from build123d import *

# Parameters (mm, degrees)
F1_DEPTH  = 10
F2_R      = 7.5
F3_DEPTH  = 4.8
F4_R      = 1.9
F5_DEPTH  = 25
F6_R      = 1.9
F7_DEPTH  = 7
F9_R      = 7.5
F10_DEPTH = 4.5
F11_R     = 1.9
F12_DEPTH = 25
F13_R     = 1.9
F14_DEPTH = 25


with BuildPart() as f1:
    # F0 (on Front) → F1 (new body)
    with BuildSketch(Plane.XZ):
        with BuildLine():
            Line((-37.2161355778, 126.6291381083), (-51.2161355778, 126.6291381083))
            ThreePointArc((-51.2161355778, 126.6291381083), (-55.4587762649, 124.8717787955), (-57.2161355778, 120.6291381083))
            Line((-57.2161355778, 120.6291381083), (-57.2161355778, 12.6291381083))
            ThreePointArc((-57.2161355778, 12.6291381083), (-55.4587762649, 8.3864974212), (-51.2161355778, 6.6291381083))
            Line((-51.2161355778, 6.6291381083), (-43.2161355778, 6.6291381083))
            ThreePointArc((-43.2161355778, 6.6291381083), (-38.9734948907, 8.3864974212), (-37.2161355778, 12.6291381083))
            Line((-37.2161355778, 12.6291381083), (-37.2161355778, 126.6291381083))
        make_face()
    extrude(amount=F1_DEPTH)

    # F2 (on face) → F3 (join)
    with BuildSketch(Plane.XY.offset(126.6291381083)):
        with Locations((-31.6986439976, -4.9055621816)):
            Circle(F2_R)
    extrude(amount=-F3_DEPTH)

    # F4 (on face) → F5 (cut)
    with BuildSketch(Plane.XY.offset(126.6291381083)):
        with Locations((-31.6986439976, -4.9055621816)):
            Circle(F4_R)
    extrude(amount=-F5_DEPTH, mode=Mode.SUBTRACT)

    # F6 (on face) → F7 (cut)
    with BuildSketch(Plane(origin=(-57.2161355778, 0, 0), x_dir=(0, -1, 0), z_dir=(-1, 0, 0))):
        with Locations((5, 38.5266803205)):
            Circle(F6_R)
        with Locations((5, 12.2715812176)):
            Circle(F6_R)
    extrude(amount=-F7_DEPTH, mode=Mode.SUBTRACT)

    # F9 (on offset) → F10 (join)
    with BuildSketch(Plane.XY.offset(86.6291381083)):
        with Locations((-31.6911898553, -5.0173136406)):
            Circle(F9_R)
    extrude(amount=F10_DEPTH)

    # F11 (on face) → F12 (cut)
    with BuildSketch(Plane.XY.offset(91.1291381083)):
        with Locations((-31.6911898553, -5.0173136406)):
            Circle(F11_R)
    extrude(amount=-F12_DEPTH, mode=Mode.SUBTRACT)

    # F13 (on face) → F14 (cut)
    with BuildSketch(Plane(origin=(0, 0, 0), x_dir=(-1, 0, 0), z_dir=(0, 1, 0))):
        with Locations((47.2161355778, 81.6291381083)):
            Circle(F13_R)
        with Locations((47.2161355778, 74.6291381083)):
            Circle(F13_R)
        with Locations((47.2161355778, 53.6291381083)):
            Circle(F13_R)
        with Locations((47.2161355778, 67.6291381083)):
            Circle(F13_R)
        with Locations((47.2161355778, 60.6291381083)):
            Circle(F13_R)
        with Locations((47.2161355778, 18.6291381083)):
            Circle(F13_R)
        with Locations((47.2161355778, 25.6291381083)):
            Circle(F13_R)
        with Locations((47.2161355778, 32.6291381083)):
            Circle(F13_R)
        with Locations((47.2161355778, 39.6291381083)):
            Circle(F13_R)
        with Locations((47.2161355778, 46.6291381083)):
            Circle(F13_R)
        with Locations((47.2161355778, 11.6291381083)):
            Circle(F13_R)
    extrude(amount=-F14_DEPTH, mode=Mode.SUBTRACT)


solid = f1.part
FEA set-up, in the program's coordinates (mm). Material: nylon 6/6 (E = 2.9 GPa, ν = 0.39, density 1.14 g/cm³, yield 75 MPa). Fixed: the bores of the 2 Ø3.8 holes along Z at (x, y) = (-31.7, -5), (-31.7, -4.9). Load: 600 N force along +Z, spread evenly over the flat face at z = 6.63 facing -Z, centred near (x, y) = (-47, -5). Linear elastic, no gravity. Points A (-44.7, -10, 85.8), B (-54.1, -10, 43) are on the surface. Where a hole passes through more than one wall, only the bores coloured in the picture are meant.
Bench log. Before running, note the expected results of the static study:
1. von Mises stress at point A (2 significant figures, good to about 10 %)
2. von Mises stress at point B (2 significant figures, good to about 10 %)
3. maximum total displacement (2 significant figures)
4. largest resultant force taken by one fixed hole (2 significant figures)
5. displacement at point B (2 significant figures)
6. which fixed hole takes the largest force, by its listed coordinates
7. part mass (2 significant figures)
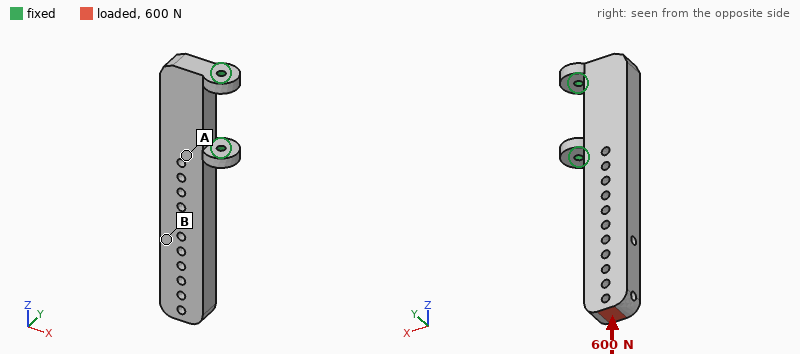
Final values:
2.5 MPa
4.6 MPa
0.34 mm
380 N
0.22 mm
(-31.7, -5)
27 g
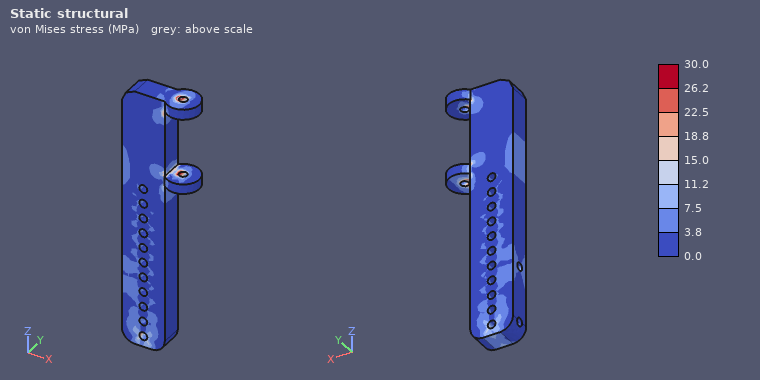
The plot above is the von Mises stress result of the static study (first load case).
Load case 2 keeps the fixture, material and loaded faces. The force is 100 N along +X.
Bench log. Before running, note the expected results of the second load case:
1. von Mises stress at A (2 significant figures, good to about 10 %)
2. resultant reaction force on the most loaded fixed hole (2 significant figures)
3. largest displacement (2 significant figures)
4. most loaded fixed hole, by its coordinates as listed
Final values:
2.3 MPa
350 N
1.5 mm
(-31.7, -5)
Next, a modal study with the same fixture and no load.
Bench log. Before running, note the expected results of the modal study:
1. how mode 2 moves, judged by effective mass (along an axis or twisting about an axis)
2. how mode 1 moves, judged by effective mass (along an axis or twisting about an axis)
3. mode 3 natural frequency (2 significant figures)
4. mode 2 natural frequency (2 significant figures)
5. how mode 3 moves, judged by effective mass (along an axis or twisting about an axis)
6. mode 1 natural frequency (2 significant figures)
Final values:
along X
along Y
1100 Hz
610 Hz
along Y
290 Hz
